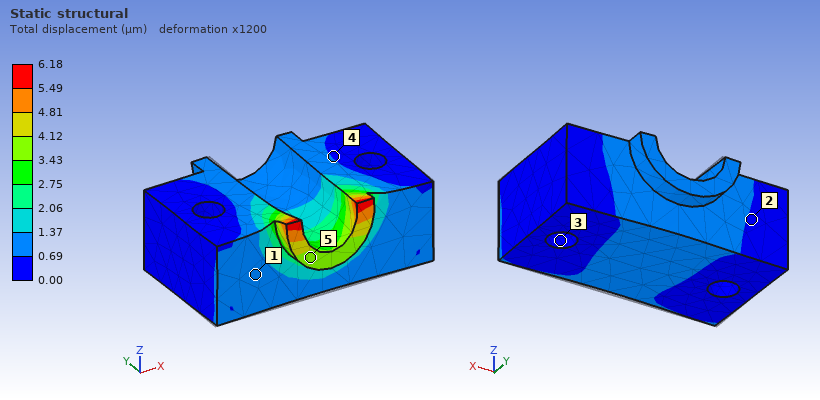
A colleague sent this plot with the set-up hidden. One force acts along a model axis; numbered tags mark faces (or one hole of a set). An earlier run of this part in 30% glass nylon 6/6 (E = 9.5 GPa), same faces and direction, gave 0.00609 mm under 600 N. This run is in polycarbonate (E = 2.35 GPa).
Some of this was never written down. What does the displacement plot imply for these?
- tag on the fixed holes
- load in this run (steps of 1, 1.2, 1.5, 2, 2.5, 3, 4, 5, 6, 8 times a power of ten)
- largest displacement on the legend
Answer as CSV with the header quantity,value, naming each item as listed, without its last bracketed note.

quantity,value
tag on the fixed holes,3
load in this run,150 N
largest displacement on the legend,6.18 µm
